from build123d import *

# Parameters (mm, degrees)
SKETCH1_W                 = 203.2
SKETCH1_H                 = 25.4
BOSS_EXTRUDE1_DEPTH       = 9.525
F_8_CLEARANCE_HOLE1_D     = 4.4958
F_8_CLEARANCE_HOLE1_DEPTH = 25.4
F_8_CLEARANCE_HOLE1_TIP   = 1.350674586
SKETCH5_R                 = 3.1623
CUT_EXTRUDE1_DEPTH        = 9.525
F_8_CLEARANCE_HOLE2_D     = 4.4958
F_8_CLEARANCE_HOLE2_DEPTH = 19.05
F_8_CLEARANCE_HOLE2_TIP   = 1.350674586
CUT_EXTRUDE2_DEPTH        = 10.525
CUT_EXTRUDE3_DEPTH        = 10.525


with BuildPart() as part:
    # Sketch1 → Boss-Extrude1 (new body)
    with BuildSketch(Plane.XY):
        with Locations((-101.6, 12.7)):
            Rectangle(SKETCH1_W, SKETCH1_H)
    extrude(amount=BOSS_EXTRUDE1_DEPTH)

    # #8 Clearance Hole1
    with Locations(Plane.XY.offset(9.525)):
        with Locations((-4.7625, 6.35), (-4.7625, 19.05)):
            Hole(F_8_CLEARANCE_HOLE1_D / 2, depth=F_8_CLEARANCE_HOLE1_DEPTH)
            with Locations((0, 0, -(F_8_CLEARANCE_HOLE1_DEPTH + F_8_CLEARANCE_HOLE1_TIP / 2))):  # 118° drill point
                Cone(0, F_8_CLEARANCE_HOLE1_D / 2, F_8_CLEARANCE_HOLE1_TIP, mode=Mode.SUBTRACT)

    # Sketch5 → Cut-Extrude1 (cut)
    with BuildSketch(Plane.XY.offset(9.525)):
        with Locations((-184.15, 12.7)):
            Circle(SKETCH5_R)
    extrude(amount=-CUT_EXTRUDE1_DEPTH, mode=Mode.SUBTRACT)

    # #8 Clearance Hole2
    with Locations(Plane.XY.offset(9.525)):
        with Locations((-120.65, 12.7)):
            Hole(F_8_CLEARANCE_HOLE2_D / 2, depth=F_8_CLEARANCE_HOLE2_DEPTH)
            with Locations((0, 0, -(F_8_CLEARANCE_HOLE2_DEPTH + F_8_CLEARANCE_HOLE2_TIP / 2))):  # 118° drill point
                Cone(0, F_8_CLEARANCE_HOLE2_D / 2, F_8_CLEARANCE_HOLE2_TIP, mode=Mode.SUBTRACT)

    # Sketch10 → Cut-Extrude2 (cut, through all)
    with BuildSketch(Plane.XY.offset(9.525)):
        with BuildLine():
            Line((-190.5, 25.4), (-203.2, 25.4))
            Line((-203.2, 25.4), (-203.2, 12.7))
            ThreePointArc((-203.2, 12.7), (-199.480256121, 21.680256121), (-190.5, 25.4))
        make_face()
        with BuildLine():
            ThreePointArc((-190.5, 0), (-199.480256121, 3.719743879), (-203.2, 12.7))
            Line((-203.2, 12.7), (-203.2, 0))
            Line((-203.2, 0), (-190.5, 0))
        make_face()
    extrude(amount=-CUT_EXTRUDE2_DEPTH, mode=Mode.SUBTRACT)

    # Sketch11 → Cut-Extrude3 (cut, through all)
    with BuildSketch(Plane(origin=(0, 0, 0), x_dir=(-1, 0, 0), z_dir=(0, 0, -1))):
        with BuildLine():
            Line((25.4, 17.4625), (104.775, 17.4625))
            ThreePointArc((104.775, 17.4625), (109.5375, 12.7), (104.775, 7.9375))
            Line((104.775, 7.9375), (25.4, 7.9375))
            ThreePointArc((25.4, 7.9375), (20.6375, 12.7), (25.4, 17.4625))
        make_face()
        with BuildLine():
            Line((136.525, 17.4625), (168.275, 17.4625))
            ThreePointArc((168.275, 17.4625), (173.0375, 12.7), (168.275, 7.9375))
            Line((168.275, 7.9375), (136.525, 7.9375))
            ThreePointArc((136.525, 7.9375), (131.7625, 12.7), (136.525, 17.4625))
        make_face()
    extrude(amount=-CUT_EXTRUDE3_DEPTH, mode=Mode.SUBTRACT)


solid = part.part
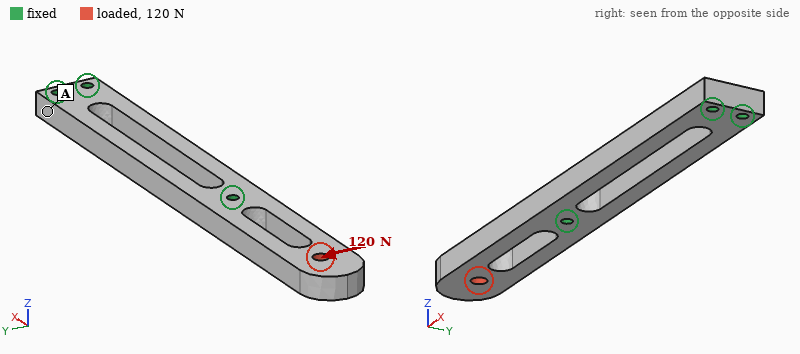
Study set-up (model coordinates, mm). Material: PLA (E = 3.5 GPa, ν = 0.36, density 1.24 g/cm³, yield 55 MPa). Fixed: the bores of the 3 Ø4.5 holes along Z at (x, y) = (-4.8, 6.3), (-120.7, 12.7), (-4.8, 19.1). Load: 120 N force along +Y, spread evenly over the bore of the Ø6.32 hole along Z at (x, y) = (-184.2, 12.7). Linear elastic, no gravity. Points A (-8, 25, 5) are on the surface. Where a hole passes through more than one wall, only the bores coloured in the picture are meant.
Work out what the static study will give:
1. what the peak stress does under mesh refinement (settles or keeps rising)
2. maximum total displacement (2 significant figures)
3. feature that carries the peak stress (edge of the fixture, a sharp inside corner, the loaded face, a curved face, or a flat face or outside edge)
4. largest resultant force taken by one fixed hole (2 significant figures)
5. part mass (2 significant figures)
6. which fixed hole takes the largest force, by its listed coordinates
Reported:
keeps rising
1.1 mm
edge of the fixture
130 N
45 g
(-120.7, 12.7)
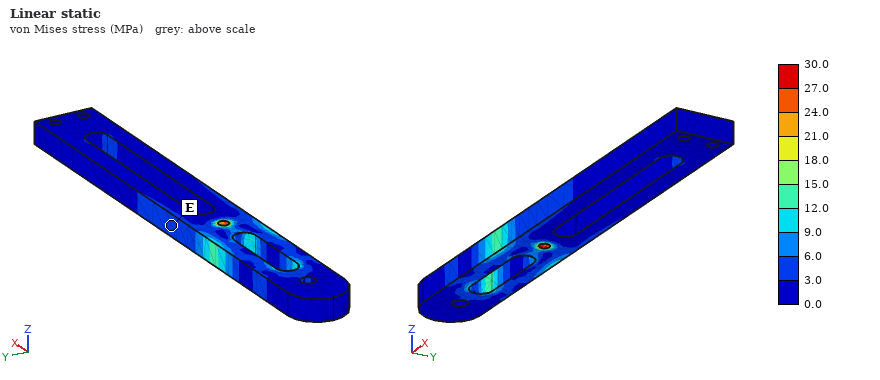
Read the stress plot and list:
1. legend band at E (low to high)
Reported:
3.0 to 6.0 MPa
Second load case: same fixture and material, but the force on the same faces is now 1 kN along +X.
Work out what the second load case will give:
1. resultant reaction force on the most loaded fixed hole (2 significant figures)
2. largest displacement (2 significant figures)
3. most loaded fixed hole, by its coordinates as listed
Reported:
940 N
0.14 mm
(-120.7, 12.7)
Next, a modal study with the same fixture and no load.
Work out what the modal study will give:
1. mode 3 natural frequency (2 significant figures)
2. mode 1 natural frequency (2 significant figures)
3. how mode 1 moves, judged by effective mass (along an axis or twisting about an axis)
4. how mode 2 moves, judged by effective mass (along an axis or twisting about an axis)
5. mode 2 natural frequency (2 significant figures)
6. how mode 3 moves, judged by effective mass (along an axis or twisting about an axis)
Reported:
1300 Hz
350 Hz
along Z
along Y
550 Hz
along Z
